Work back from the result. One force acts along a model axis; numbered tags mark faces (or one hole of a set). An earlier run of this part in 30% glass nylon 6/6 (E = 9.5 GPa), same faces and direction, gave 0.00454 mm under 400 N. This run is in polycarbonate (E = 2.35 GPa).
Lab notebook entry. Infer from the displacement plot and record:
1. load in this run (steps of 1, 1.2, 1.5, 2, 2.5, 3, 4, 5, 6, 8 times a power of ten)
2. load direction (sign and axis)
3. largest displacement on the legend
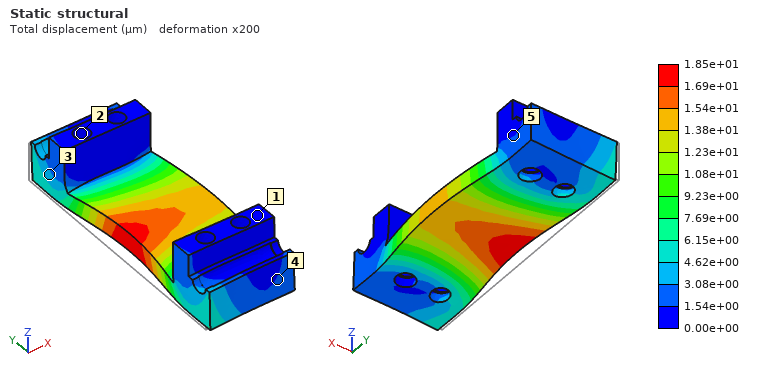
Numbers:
400 N
+X
1.85e+01 µm
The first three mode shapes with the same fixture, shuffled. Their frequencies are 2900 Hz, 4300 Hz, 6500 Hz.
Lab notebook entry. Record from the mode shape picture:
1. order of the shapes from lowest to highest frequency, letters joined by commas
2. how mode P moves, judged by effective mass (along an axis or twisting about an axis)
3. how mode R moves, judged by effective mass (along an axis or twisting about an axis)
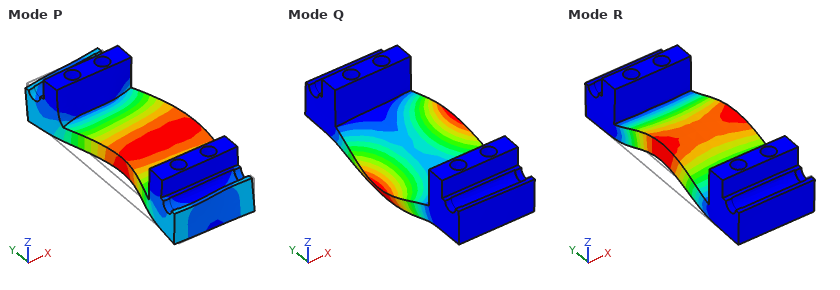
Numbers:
R, Q, P
along X
along Z
